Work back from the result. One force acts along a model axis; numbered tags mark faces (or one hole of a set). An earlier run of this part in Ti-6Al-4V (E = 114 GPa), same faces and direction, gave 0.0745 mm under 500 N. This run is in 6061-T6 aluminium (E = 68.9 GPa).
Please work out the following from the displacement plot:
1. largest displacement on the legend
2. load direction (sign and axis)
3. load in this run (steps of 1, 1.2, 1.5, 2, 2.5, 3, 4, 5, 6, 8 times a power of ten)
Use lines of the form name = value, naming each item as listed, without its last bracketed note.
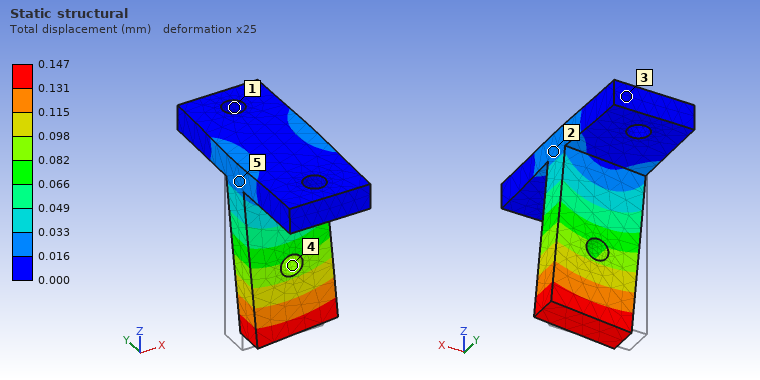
largest displacement on the legend = 0.147 mm
load direction = +X
load in this run = 600 N
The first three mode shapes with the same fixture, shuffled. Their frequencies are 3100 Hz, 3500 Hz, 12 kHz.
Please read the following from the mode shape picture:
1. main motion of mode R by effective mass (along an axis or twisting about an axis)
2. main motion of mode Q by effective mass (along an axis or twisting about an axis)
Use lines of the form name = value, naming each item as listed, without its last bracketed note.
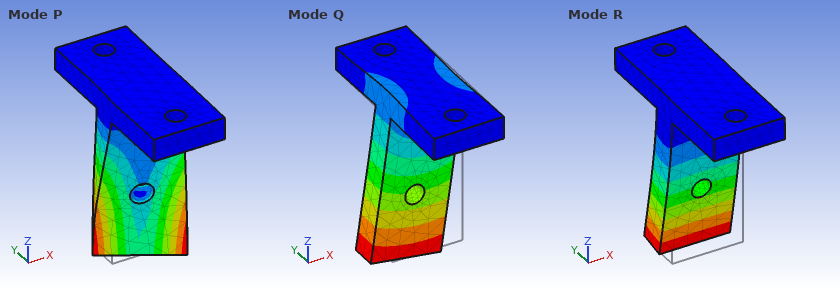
main motion of mode R by effective mass = along Y
main motion of mode Q by effective mass = along X
